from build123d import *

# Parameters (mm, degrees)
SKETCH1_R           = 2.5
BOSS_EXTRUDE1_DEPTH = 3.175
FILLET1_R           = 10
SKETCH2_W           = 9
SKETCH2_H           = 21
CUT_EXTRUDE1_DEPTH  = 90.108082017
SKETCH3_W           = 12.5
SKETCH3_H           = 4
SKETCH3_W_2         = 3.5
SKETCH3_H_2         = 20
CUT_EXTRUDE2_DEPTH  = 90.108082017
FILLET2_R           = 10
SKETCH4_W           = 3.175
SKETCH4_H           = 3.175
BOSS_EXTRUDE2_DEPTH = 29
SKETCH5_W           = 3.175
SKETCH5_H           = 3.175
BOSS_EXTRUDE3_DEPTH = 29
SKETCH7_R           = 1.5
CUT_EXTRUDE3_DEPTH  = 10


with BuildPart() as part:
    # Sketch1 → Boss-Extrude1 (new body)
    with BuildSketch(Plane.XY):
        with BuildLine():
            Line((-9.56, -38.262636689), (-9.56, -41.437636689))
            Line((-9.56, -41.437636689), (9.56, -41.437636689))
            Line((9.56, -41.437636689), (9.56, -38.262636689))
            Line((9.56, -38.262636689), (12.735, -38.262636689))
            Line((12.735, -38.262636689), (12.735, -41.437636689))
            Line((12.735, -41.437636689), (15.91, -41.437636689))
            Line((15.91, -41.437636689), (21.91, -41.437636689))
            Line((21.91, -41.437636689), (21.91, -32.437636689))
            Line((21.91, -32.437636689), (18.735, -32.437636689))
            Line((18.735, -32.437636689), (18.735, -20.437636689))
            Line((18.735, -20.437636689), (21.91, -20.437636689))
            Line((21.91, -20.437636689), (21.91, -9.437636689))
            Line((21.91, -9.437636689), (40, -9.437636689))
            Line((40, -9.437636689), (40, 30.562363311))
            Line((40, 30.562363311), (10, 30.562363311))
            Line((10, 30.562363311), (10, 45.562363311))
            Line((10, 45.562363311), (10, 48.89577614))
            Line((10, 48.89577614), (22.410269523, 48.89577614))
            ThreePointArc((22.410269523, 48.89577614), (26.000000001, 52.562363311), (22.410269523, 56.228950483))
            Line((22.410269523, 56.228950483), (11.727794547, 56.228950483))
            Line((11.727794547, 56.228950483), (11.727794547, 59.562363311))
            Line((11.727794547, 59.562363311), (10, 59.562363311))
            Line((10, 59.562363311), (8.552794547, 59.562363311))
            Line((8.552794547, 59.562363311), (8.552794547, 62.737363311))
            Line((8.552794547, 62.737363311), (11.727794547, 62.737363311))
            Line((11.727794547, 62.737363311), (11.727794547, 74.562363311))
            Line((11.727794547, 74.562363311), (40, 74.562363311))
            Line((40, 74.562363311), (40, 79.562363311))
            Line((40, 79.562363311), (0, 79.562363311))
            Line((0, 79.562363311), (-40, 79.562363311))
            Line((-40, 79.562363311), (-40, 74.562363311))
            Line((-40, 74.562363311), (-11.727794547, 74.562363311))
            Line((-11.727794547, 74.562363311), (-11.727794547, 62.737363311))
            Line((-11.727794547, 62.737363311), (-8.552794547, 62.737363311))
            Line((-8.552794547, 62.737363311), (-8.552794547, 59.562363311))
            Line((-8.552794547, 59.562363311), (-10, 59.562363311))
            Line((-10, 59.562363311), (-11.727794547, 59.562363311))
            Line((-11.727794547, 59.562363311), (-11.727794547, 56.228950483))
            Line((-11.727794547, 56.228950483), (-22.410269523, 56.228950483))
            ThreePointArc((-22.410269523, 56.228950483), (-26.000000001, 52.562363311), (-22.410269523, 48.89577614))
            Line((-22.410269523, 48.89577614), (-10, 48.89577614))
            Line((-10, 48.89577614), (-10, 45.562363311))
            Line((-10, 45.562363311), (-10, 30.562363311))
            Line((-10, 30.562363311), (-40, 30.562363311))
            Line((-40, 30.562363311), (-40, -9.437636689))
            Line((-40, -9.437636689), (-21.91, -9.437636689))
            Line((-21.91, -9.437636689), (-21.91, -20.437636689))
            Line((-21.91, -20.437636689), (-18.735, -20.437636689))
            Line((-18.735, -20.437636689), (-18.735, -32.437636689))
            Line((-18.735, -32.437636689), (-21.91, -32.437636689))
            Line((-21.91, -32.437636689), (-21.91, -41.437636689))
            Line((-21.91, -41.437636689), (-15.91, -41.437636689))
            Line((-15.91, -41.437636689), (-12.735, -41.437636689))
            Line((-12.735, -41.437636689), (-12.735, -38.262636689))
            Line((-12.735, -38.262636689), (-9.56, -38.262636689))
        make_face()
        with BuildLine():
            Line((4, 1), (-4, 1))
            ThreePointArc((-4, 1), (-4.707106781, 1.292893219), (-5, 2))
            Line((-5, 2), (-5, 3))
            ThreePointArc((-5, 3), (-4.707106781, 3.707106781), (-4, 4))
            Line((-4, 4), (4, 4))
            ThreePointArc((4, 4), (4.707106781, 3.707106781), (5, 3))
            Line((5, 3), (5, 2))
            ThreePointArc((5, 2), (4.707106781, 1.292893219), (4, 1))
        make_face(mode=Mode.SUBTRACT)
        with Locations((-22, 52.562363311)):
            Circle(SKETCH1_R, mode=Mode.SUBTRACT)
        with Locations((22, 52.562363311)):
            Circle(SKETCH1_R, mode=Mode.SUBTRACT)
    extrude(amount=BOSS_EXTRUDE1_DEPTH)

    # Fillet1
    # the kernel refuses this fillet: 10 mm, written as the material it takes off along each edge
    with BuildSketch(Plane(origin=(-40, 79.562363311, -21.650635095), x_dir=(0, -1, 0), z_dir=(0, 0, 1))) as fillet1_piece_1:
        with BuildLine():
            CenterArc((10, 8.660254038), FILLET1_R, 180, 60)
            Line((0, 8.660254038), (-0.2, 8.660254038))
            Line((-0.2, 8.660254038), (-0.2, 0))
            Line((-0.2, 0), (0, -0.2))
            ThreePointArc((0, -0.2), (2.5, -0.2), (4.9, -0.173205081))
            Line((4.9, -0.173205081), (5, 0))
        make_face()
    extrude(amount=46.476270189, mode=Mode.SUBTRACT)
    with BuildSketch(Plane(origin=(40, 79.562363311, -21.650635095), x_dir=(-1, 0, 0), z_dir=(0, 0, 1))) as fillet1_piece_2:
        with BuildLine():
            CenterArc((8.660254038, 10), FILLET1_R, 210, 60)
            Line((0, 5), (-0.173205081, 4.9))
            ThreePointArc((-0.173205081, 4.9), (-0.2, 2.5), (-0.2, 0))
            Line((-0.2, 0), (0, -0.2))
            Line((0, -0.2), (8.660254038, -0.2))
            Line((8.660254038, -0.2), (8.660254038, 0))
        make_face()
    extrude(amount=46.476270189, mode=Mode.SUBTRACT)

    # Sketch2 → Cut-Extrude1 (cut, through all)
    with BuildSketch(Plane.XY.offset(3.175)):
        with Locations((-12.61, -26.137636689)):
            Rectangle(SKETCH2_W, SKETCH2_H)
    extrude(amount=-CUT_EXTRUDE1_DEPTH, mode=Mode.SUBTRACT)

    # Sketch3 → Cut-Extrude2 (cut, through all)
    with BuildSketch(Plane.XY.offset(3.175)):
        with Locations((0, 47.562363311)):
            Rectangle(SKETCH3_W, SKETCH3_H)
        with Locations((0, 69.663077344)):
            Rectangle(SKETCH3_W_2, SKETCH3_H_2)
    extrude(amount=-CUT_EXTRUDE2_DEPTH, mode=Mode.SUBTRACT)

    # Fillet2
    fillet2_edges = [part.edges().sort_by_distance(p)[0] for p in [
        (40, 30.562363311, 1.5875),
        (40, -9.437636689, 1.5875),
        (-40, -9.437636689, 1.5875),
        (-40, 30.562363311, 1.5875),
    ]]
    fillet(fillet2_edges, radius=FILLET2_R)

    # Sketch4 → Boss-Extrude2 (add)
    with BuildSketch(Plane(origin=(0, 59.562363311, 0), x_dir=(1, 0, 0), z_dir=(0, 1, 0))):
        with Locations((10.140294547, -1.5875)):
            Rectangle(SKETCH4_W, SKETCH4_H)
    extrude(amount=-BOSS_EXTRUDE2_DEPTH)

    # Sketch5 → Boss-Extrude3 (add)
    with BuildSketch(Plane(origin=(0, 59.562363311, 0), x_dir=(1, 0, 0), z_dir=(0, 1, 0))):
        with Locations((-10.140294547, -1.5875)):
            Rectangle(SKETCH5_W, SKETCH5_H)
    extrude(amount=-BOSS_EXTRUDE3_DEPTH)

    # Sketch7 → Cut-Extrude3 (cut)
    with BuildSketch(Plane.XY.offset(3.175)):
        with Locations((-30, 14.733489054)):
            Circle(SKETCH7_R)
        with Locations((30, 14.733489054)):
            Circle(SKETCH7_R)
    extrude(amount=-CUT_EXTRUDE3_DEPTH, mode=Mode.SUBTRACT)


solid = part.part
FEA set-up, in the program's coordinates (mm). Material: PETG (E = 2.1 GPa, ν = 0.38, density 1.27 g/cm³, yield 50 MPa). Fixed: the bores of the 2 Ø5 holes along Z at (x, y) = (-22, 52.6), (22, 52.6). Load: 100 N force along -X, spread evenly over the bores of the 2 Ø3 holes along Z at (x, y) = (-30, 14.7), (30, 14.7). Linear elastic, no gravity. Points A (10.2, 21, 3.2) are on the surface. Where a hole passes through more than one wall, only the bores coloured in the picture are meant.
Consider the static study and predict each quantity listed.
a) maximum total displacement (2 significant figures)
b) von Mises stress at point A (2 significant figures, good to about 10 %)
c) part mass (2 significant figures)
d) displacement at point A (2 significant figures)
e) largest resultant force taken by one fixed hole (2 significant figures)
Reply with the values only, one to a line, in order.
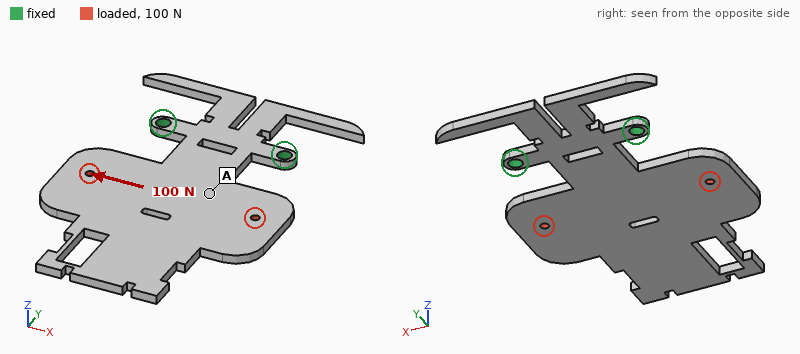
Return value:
1.7 mm
1.8 MPa
23 g
0.51 mm
120 N
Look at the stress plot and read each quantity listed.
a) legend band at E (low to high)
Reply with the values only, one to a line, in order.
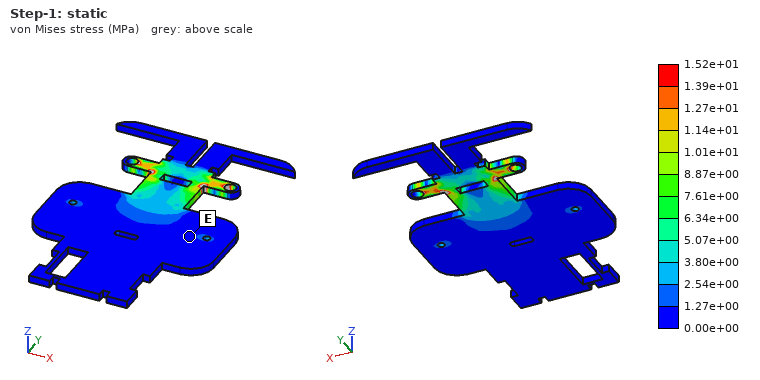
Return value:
0.00e+00 to 1.27e+00 MPa
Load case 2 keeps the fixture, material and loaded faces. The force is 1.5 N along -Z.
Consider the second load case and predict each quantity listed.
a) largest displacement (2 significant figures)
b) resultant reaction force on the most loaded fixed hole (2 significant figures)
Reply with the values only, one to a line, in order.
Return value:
1.4 mm
0.75 N
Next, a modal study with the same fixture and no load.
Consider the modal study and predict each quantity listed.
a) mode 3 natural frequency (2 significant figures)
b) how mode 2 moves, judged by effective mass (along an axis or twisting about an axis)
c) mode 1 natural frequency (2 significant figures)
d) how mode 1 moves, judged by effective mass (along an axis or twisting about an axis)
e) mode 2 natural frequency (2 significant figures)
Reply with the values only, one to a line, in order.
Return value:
280 Hz
twisting about Y
42 Hz
along Z
140 Hz
